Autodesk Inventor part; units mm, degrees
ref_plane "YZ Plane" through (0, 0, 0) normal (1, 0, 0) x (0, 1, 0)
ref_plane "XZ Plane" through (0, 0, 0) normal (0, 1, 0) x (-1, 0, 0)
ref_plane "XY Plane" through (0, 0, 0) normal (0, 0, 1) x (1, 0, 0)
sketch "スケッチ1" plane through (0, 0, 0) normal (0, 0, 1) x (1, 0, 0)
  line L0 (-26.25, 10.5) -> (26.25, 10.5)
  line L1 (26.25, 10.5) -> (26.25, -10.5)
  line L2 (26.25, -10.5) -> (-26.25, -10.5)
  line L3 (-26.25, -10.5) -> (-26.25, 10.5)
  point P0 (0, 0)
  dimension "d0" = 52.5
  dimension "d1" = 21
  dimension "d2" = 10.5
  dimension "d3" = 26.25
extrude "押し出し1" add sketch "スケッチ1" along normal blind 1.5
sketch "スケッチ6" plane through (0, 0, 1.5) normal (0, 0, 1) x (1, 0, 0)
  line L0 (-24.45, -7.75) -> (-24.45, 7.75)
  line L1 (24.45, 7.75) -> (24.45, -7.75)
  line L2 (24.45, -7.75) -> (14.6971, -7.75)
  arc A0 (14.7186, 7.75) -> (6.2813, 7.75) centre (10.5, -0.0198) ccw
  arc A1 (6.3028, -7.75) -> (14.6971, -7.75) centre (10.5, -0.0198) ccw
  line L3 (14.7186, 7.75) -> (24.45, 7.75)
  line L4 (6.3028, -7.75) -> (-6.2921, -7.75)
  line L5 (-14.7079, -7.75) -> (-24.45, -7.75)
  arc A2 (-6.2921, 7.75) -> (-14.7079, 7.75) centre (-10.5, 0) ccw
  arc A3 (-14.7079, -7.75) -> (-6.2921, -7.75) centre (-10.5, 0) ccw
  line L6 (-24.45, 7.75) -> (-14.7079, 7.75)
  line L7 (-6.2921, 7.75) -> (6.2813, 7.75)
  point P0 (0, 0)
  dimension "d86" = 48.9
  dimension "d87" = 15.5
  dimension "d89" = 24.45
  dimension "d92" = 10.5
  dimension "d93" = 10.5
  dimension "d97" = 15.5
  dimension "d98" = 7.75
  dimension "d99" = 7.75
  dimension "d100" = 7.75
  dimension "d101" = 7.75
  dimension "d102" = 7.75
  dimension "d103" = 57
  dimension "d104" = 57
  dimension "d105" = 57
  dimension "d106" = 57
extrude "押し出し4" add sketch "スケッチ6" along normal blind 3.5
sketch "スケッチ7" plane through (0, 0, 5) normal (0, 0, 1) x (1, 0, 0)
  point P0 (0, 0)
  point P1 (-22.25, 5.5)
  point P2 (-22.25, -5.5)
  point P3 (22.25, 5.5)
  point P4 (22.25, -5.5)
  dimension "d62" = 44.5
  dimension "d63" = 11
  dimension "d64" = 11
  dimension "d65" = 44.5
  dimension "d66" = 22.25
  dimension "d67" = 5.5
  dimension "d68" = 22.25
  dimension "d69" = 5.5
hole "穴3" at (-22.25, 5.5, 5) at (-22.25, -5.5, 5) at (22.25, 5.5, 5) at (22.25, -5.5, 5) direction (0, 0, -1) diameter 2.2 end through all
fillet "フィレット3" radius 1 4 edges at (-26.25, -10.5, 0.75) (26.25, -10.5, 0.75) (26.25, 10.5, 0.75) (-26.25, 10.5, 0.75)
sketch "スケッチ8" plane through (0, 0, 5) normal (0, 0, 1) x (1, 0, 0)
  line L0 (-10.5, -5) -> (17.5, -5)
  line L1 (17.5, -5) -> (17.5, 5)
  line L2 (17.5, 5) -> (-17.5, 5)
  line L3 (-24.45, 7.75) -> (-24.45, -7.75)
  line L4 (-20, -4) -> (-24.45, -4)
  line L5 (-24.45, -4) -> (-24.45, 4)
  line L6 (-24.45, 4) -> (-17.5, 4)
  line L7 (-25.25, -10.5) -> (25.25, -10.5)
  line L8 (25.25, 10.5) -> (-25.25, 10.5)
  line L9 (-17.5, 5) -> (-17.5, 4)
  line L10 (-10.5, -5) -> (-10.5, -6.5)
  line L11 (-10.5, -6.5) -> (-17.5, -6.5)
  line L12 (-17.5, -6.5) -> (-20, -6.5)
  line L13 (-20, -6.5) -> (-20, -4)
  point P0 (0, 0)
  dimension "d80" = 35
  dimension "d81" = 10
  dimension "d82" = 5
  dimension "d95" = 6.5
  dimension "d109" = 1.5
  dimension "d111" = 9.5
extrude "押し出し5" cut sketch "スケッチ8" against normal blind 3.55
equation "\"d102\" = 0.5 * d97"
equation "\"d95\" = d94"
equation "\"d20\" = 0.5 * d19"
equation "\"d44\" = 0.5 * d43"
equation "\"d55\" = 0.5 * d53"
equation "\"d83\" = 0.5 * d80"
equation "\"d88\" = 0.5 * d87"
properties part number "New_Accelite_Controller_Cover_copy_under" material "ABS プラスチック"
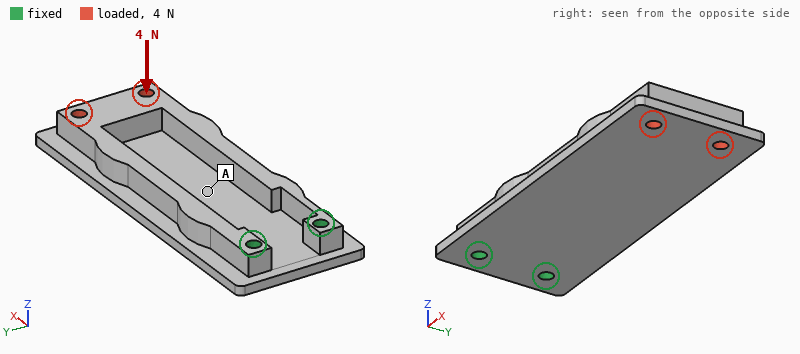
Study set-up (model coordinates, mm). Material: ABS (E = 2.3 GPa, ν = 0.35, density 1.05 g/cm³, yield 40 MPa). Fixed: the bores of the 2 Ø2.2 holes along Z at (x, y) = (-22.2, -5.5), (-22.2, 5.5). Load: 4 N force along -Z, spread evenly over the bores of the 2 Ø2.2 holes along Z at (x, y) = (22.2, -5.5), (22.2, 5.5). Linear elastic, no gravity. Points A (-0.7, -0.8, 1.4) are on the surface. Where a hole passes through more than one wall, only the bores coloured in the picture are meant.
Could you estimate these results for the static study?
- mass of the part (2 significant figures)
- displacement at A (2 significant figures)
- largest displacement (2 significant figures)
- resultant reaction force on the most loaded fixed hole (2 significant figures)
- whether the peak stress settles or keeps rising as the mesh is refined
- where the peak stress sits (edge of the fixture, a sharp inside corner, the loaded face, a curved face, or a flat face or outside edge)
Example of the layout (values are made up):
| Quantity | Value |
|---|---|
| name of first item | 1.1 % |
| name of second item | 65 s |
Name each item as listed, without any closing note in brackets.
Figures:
| Quantity | Value |
|---|---|
| mass of the part | 3.0 g |
| displacement at A | 0.18 mm |
| largest displacement | 0.68 mm |
| resultant reaction force on the most loaded fixed hole | 4.7 N |
| whether the peak stress settles or keeps rising as the mesh is refined | keeps rising |
| where the peak stress sits | a sharp inside corner |
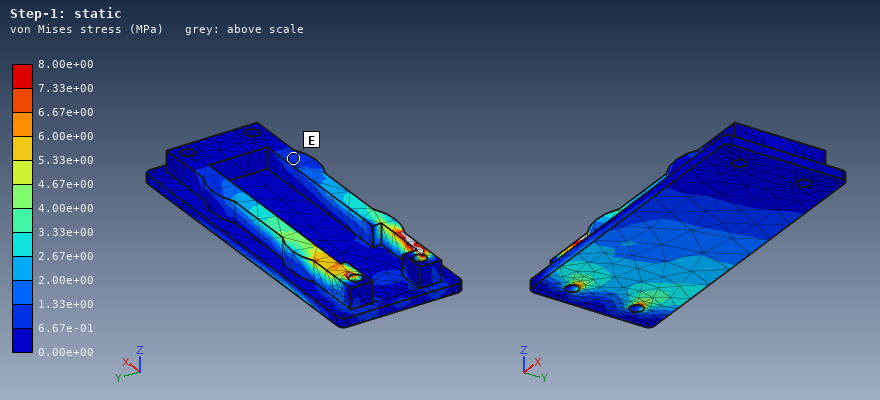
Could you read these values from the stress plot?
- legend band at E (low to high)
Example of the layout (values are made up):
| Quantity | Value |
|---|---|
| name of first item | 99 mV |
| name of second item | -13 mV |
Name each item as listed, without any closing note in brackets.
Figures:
| Quantity | Value |
|---|---|
| legend band at E | 6.67e-01 to 1.33e+00 MPa |
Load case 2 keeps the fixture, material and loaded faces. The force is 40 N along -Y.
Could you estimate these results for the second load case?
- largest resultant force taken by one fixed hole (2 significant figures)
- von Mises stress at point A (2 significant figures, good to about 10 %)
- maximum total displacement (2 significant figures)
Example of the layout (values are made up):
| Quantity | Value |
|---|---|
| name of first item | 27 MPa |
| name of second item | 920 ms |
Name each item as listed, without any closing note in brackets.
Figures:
| Quantity | Value |
|---|---|
| largest resultant force taken by one fixed hole | 140 N |
| von Mises stress at point A | 5.6 MPa |
| maximum total displacement | 0.66 mm |
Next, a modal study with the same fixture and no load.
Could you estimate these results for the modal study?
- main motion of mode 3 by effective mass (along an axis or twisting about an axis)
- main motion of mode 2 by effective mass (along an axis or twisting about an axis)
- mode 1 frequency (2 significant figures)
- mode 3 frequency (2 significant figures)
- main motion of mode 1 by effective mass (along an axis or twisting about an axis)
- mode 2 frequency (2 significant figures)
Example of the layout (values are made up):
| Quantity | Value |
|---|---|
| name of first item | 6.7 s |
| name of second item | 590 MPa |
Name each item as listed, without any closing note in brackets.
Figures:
| Quantity | Value |
|---|---|
| main motion of mode 3 by effective mass | along Y |
| main motion of mode 2 by effective mass | along Y |
| mode 1 frequency | 420 Hz |
| mode 3 frequency | 1700 Hz |
| main motion of mode 1 by effective mass | along Z |
| mode 2 frequency | 1100 Hz |
